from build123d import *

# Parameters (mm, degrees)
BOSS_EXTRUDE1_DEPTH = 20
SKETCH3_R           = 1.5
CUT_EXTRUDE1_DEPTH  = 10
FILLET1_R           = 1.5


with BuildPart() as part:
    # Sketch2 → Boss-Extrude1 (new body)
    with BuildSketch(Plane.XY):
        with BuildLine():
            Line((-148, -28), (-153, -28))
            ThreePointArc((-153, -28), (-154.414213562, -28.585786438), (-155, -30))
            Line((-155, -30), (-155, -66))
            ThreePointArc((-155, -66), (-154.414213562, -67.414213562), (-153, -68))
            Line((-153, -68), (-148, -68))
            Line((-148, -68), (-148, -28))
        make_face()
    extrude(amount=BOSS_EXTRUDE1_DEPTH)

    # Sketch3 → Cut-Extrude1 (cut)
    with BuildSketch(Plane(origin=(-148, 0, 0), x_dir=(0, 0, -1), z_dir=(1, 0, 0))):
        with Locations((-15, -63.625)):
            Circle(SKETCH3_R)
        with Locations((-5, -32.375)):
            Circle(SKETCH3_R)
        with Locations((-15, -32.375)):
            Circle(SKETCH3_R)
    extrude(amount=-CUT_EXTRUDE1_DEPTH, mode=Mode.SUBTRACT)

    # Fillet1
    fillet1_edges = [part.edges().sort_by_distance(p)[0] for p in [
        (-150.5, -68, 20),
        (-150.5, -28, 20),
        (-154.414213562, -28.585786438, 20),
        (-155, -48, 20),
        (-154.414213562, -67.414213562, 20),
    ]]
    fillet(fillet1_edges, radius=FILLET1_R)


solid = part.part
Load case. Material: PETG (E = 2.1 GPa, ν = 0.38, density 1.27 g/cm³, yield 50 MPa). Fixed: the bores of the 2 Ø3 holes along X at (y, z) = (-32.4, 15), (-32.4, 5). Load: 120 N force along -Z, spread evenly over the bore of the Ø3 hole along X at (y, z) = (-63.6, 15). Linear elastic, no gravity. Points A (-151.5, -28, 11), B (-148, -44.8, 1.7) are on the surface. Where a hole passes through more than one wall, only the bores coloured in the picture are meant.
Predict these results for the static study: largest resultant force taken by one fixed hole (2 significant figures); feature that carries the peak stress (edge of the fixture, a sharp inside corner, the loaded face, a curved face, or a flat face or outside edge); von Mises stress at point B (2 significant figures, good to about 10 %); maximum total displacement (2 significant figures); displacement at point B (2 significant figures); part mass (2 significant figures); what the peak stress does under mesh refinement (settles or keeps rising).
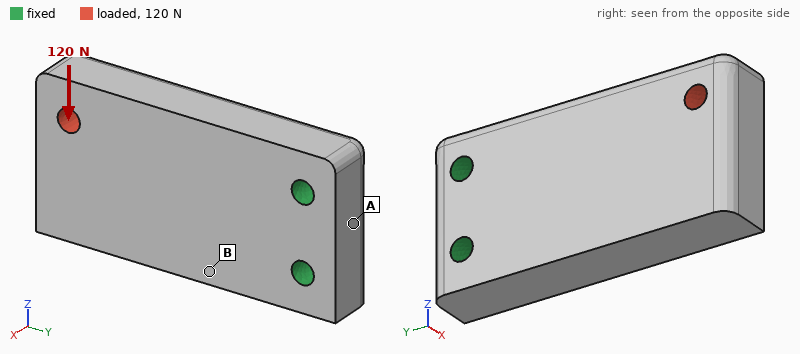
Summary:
310 N
edge of the fixture
4.1 MPa
0.23 mm
0.067 mm
6.8 g
keeps rising
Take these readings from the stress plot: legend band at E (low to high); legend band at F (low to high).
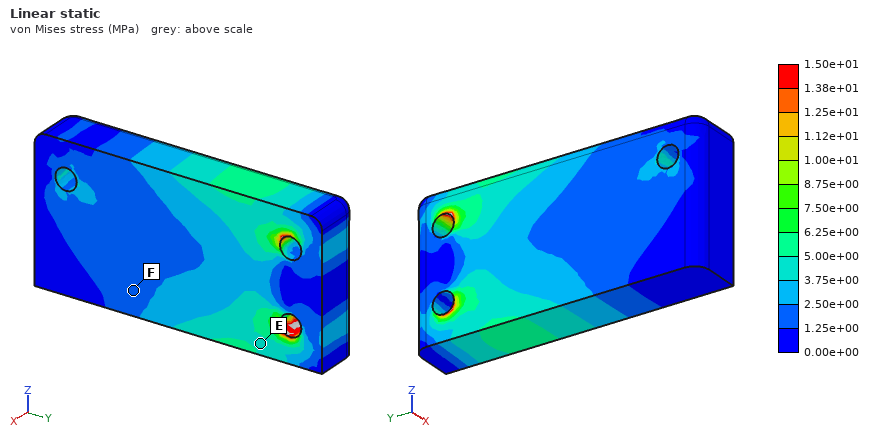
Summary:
3.75e+00 to 5.00e+00 MPa
1.25e+00 to 2.50e+00 MPa
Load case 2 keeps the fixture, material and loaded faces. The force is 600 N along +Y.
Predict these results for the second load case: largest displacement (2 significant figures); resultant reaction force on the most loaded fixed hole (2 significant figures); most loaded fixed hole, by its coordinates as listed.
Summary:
0.25 mm
560 N
(-32.4, 15)
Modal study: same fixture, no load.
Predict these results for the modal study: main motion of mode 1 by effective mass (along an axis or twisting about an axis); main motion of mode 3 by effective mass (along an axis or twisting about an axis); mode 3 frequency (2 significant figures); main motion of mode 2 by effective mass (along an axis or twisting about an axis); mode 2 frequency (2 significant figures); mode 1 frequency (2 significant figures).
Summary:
along X
twisting about Y
3600 Hz
along Z
2500 Hz
1100 Hz
